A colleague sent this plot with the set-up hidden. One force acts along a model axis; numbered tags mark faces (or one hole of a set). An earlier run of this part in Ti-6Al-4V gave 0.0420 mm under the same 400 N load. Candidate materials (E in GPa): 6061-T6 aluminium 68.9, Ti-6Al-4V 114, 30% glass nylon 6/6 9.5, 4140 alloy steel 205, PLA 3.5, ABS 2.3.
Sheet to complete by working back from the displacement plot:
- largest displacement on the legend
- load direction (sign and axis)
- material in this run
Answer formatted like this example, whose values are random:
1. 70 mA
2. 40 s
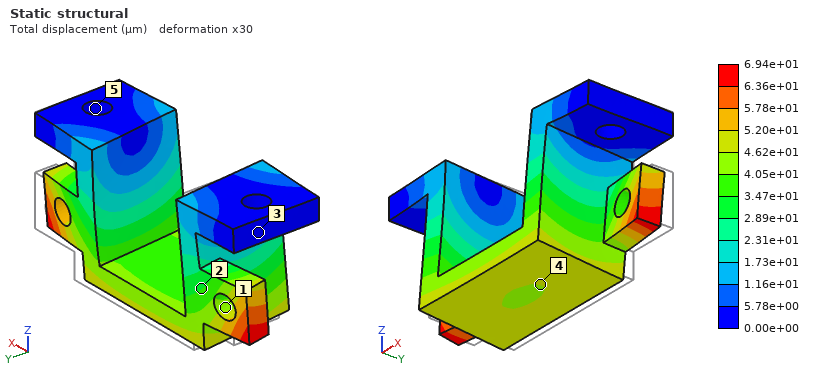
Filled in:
1. 6.94e+01 µm
2. -Y
3. 6061-T6 aluminium
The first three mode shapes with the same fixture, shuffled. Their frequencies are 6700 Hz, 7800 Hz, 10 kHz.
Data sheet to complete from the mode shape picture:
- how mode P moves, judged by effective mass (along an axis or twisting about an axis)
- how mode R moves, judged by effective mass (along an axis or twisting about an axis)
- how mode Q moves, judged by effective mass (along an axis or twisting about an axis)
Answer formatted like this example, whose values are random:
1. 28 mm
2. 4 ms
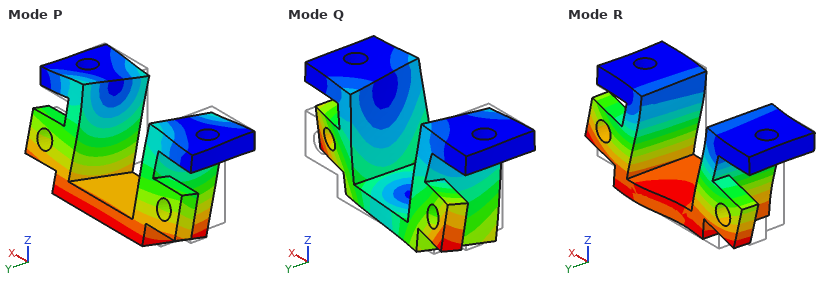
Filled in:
1. along Y
2. along X
3. twisting about Z
